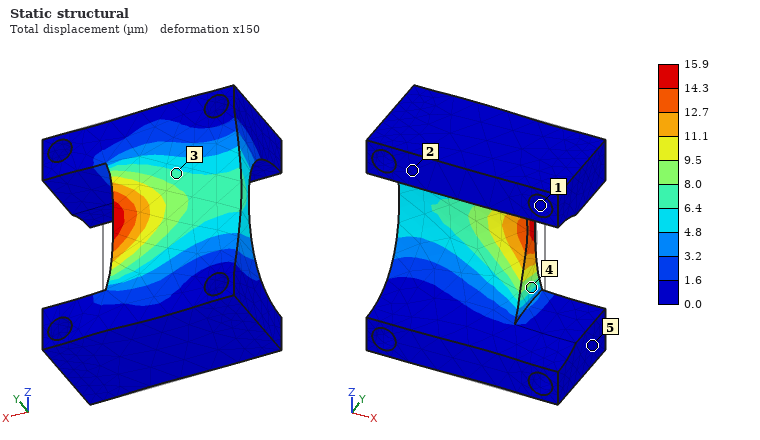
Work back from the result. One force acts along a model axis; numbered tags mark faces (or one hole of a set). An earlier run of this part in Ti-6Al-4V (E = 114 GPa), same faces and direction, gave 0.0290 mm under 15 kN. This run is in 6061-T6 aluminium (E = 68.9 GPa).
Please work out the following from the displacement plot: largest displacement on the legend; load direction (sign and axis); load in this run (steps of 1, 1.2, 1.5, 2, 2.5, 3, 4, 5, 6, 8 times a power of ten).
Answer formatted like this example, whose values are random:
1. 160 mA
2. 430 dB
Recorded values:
1. 15.9 µm
2. -X
3. 5 kN
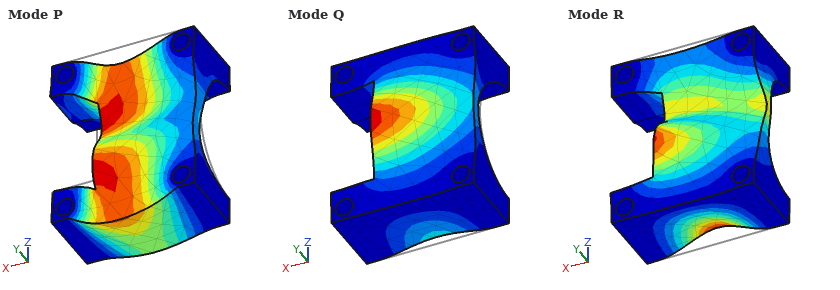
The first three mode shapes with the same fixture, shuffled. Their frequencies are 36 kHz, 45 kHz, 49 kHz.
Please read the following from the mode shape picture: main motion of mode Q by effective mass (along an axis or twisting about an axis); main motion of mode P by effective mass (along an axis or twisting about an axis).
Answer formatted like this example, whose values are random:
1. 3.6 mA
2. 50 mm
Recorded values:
1. along Y
2. along Z
